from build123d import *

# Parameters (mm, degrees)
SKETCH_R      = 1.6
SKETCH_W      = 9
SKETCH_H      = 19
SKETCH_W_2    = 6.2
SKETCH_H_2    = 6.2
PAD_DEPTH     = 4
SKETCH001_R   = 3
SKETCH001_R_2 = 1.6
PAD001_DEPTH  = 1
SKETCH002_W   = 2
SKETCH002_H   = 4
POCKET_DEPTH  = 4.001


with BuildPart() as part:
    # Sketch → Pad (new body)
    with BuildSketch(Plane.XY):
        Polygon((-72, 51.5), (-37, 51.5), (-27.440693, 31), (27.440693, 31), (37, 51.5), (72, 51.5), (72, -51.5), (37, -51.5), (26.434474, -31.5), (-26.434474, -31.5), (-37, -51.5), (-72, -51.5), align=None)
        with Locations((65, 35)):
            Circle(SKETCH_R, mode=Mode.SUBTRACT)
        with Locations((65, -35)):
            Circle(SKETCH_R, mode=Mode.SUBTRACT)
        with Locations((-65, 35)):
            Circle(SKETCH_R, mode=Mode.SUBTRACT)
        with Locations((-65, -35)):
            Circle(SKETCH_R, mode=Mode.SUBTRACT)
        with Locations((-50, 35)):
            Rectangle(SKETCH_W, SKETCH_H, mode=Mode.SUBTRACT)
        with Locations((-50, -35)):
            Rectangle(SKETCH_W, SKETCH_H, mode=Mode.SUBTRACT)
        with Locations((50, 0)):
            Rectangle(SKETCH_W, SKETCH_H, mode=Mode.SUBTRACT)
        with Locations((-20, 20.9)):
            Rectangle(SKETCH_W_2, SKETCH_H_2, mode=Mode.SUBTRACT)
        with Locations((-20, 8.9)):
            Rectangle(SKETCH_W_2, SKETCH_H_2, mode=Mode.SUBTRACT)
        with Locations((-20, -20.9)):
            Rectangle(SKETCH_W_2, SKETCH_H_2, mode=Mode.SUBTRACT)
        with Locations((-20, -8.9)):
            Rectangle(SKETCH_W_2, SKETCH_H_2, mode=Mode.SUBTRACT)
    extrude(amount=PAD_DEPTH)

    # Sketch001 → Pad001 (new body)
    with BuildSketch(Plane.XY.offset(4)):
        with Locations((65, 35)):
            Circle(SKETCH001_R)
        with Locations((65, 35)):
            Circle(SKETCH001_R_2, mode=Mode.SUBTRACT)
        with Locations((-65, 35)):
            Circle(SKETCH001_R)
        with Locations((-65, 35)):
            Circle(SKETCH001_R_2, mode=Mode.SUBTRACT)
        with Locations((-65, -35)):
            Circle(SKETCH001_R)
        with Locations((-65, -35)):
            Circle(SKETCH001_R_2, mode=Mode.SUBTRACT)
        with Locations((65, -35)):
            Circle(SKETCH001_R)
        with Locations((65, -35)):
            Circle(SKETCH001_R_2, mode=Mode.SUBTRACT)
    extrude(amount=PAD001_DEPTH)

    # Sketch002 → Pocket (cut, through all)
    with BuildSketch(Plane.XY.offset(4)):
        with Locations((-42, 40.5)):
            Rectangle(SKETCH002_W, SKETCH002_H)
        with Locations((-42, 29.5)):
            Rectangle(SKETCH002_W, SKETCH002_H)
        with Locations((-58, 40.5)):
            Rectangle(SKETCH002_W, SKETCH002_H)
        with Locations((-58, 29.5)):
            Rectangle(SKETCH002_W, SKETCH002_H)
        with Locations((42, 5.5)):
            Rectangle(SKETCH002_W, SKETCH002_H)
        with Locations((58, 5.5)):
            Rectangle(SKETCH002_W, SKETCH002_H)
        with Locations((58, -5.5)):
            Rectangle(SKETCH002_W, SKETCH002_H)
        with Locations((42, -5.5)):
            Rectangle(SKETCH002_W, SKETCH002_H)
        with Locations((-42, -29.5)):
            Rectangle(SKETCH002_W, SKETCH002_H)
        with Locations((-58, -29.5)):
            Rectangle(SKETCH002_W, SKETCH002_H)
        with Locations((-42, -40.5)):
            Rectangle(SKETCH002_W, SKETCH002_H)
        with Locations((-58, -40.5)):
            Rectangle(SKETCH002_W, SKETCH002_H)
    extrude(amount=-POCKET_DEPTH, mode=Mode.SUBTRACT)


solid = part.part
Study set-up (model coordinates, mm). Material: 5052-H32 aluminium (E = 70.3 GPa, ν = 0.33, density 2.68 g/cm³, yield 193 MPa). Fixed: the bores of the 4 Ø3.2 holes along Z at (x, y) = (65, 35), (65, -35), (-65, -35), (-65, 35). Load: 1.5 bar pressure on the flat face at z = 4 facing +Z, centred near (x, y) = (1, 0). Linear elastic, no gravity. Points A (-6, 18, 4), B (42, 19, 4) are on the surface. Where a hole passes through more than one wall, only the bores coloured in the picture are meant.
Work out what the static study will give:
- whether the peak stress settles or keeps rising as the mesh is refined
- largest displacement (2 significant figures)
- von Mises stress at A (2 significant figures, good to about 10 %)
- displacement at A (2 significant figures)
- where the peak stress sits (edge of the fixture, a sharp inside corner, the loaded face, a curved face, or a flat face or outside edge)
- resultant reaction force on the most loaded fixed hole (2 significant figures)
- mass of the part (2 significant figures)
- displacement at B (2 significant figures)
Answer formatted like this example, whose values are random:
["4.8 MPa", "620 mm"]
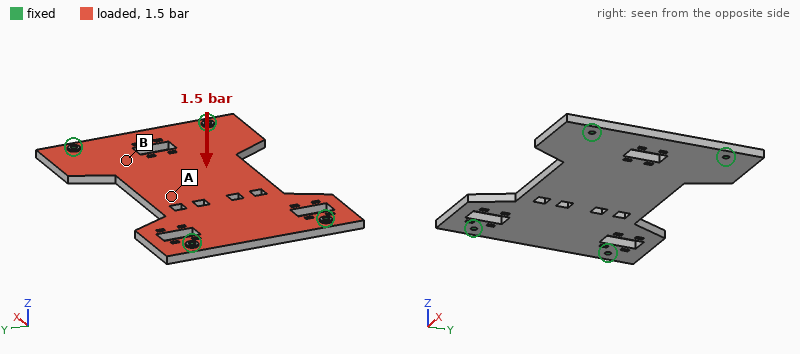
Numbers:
["keeps rising", "0.43 mm", "40 MPa", "0.42 mm", "edge of the fixture", "450 N", "120 g", "0.18 mm"]
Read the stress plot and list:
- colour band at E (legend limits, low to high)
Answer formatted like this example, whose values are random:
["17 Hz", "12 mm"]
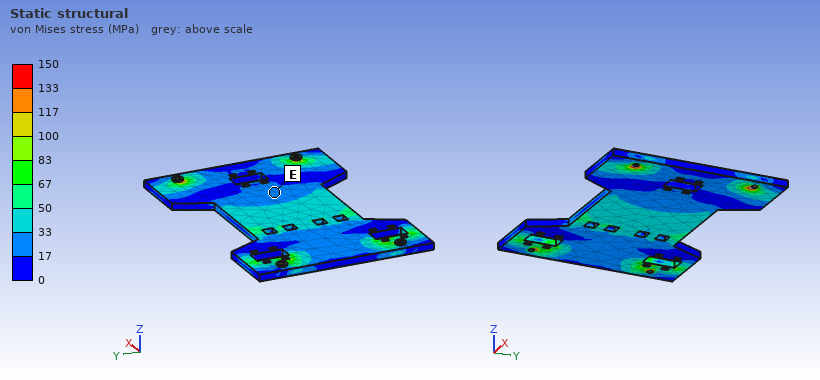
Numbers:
["17 to 33 MPa"]
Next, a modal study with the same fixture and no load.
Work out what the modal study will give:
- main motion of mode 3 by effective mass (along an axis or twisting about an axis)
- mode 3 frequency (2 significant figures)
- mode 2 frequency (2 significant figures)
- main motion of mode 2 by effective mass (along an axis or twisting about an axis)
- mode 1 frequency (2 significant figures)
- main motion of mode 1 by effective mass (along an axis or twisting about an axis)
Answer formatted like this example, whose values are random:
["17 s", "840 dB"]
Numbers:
["twisting about Y", "2600 Hz", "2100 Hz", "twisting about X", "1100 Hz", "along Z"]
